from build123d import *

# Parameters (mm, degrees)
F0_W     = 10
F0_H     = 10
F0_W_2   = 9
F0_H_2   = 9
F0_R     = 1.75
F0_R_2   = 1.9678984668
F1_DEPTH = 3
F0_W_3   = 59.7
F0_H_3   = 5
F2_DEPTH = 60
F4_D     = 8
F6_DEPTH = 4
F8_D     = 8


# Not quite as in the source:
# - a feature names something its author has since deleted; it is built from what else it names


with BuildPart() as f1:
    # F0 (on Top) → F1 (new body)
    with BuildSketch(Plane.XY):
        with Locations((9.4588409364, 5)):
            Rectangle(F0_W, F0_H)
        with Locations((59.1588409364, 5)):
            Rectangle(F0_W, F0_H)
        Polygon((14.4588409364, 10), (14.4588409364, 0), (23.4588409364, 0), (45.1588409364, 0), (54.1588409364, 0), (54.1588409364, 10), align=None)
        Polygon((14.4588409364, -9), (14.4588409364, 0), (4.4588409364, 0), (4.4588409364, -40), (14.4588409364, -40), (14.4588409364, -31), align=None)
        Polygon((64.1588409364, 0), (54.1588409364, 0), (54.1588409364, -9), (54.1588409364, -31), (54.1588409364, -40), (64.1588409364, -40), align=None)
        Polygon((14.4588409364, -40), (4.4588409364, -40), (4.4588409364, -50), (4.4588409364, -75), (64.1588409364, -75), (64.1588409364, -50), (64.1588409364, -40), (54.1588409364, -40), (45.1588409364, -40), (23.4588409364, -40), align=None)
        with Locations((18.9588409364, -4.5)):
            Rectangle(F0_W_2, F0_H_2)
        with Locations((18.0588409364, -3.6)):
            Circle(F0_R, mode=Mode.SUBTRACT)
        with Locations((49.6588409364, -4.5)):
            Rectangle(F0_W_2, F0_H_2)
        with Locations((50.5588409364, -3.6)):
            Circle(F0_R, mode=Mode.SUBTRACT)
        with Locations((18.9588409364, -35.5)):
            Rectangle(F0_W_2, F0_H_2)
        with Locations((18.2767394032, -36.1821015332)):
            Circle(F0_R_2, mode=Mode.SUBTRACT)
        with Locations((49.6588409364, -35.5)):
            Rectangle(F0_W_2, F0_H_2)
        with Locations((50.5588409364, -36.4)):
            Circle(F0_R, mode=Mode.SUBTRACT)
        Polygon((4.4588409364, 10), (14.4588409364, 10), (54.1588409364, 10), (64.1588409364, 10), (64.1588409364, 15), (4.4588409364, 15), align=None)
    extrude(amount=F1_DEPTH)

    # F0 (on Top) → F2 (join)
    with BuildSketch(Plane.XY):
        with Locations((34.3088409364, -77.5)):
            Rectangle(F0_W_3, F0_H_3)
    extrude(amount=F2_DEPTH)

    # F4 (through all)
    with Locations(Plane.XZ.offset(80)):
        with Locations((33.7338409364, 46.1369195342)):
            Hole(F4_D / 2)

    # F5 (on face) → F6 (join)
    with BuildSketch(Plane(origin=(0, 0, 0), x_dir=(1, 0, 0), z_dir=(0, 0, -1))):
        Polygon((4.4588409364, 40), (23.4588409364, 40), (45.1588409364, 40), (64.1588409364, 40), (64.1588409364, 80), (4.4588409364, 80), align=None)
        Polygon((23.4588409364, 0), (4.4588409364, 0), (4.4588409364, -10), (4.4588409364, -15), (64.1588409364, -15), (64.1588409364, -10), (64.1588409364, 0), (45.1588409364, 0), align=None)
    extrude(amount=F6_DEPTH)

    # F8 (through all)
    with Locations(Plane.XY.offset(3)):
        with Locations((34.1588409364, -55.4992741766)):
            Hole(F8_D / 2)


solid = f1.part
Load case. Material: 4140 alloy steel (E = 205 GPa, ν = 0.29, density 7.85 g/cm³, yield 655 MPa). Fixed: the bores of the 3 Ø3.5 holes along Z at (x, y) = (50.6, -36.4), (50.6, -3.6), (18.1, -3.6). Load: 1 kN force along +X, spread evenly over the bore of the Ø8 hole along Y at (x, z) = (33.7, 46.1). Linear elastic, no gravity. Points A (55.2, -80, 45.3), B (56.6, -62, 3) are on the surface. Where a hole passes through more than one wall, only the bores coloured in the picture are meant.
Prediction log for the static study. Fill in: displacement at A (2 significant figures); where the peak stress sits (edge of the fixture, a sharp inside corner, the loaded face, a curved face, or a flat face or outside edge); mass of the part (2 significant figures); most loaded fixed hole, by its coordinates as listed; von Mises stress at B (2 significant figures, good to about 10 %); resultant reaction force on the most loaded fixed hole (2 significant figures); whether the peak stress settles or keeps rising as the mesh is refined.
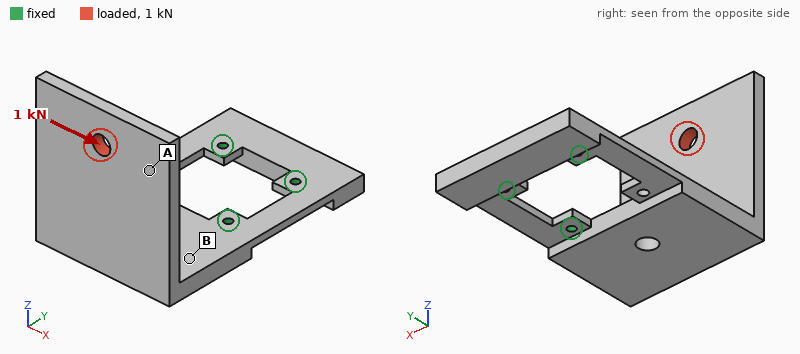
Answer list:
0.72 mm
edge of the fixture
330 g
(50.6, -36.4)
130 MPa
1.4 kN
keeps rising
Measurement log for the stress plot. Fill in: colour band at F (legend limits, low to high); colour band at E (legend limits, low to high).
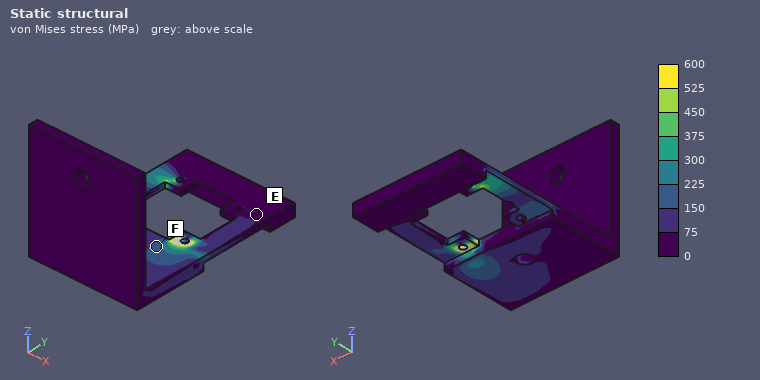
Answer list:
150 to 225 MPa
0 to 75 MPa
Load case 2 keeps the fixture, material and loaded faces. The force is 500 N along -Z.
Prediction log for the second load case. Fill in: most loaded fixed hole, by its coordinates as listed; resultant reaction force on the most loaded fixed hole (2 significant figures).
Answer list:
(50.6, -36.4)
640 N
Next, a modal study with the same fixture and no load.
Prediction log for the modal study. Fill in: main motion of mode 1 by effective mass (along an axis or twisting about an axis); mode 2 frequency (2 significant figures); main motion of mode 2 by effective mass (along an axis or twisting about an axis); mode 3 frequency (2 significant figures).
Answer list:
along Z
590 Hz
along X
1300 Hz
